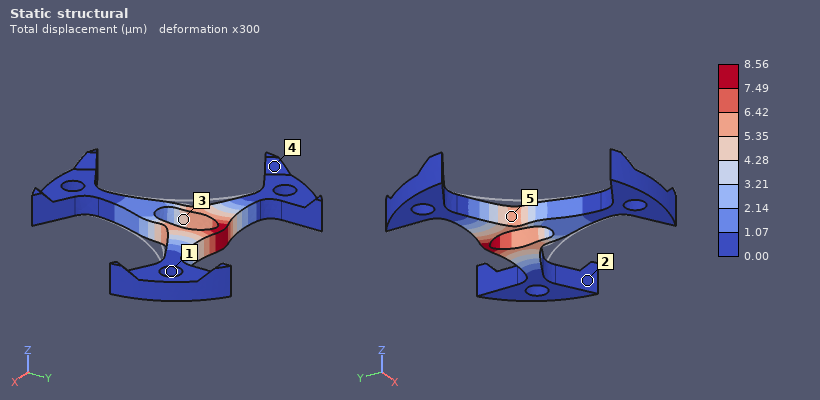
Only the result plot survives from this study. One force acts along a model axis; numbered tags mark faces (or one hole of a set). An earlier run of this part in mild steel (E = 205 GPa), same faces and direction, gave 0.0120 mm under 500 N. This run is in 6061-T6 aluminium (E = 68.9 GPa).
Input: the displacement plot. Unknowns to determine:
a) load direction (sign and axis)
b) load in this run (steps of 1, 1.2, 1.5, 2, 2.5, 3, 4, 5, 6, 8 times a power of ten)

+Y
120 N
